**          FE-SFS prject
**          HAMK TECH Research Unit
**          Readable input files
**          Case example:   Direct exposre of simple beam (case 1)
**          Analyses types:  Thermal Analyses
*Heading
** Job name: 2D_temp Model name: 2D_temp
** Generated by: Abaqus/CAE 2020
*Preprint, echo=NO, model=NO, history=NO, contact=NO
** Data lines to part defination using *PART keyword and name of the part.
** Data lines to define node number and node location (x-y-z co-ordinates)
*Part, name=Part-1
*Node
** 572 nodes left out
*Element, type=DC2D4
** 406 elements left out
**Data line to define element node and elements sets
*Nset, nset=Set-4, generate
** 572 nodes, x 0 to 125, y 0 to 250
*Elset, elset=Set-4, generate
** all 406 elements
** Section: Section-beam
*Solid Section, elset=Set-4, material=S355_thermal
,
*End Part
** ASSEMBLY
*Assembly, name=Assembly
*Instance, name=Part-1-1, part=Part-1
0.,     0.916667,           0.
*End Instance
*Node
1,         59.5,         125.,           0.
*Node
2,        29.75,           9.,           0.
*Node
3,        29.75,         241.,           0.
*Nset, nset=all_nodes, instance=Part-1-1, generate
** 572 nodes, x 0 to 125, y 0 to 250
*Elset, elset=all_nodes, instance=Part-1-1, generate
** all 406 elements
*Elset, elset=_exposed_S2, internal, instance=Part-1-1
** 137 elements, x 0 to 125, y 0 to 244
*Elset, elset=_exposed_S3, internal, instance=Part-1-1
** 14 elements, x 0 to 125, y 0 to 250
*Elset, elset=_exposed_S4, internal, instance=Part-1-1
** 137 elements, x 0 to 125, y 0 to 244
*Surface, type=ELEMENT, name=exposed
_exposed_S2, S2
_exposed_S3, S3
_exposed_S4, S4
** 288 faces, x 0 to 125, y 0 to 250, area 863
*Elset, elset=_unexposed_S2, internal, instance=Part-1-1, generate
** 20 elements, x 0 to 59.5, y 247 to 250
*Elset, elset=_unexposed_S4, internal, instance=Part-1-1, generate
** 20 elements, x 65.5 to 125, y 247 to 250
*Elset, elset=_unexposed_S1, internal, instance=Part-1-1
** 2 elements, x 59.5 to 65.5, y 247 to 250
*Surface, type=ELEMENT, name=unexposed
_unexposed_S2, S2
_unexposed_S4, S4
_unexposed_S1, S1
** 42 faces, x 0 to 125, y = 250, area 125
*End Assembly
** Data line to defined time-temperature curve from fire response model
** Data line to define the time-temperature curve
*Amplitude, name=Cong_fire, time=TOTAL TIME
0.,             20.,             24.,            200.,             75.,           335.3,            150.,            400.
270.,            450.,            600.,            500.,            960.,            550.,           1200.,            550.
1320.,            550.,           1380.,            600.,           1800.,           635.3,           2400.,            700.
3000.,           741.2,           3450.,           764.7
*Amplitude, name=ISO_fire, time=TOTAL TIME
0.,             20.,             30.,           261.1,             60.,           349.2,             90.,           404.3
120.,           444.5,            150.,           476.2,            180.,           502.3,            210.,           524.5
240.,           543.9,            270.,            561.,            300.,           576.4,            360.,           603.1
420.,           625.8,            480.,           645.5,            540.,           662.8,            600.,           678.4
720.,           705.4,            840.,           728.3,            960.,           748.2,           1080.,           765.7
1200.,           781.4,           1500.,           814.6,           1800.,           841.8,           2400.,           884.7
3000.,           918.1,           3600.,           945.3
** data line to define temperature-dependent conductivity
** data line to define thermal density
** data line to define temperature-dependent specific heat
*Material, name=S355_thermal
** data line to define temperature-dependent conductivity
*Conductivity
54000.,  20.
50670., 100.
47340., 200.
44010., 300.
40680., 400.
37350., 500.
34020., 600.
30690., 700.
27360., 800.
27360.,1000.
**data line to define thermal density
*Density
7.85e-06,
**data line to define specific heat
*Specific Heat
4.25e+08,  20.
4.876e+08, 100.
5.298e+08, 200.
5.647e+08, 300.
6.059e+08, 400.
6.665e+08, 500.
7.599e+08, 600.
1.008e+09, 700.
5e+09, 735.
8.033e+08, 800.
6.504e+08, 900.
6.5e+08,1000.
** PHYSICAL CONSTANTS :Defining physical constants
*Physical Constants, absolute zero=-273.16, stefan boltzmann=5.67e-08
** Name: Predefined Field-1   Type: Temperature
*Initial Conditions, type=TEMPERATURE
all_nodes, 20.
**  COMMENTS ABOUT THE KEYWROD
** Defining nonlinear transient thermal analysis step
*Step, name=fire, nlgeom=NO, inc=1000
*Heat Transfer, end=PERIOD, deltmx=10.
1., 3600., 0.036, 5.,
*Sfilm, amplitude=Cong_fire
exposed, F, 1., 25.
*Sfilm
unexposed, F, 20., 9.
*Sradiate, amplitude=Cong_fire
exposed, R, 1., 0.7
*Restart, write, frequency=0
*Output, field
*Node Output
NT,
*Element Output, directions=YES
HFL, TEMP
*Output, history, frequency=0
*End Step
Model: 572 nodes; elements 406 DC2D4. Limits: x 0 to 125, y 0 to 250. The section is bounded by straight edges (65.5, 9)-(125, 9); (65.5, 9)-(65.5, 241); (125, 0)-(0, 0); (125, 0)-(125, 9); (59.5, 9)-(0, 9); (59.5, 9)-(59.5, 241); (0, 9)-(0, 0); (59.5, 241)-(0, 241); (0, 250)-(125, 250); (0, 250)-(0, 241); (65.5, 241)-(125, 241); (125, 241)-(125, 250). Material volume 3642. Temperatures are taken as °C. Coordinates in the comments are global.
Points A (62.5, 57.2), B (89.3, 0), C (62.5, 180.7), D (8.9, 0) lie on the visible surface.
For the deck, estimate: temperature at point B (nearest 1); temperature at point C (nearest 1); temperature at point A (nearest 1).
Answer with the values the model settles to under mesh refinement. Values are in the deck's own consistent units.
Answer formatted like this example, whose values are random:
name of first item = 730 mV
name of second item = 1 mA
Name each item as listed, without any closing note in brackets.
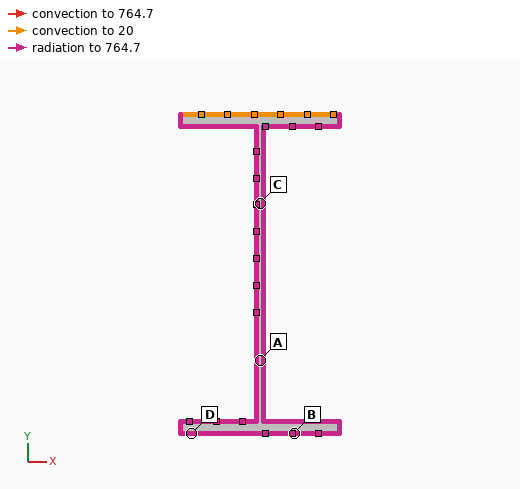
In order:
temperature at point B = 739 °C
temperature at point C = 744 °C
temperature at point A = 745 °C
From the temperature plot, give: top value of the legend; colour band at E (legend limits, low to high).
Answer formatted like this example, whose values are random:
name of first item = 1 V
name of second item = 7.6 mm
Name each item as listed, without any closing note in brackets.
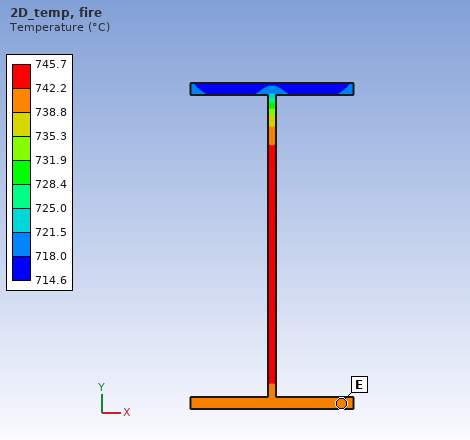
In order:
top value of the legend = 745.7 °C
colour band at E = 738.8 to 742.2 °C
